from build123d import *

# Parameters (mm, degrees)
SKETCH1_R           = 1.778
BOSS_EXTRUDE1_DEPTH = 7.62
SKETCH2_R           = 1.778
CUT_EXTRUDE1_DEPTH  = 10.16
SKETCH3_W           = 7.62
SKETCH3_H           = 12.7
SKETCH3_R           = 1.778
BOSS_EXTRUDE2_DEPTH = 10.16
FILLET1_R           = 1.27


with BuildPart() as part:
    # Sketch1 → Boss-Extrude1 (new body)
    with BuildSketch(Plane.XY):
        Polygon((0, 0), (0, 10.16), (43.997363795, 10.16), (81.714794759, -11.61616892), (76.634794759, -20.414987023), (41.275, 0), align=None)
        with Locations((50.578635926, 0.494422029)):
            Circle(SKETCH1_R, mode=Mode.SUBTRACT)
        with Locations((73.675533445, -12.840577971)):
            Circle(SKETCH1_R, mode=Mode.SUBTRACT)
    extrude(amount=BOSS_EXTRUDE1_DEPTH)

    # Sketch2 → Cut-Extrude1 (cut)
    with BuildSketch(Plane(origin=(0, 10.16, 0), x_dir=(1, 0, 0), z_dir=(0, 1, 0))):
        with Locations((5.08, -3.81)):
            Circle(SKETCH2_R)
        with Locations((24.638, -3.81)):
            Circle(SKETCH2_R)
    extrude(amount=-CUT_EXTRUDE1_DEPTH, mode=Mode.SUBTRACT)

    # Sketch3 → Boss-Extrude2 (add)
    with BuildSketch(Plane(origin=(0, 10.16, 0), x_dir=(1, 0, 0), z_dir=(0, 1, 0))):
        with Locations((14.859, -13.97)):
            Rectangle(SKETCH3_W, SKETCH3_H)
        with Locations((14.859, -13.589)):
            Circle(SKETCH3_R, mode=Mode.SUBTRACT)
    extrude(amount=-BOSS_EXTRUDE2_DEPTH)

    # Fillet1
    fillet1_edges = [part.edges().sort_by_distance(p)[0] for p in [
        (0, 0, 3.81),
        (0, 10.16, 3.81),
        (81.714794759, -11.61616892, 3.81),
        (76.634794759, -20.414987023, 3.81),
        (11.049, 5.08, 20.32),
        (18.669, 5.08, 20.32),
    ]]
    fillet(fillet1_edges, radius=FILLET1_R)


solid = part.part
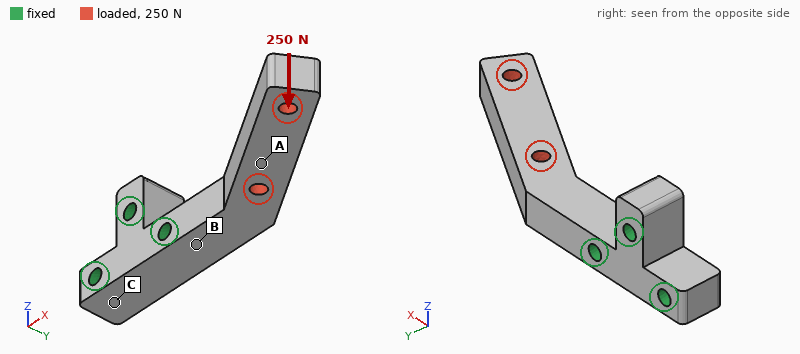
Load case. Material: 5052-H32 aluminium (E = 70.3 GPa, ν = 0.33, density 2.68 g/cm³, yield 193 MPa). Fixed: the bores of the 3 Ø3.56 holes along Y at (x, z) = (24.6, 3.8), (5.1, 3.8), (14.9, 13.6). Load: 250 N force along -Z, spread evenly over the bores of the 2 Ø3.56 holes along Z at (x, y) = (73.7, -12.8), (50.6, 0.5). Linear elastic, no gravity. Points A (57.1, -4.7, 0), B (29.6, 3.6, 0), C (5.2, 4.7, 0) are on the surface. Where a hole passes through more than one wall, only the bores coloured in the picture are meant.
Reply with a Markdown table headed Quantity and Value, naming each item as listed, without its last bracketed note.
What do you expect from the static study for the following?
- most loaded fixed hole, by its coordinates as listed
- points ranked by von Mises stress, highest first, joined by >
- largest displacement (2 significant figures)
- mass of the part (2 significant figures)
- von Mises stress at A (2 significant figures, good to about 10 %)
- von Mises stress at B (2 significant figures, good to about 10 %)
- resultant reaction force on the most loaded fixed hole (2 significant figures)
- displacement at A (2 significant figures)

| Quantity | Value |
|---|---|
| most loaded fixed hole, by its coordinates as listed | (24.6, 3.8) |
| points ranked by von Mises stress, highest first, joined by > | B > A > C |
| largest displacement | 0.40 mm |
| mass of the part | 19 g |
| von Mises stress at A | 23 MPa |
| von Mises stress at B | 88 MPa |
| resultant reaction force on the most loaded fixed hole | 450 N |
| displacement at A | 0.18 mm |
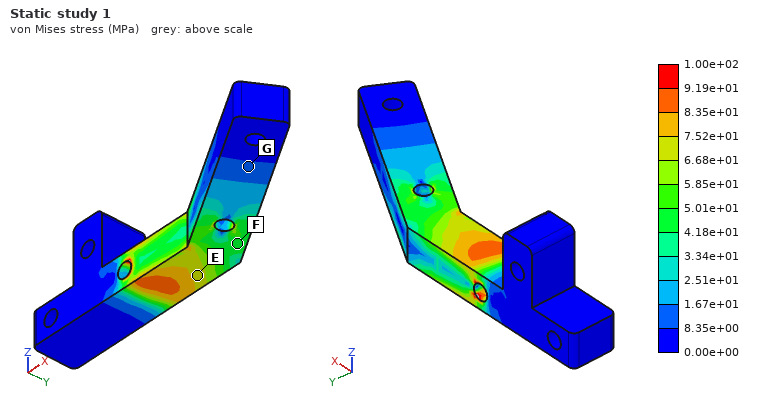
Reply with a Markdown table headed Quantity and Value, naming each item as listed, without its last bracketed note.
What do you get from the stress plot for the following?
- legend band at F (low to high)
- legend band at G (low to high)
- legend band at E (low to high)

| Quantity | Value |
|---|---|
| legend band at F | 4.18e+01 to 5.01e+01 MPa |
| legend band at G | 8.35e+00 to 1.67e+01 MPa |
| legend band at E | 6.68e+01 to 7.52e+01 MPa |
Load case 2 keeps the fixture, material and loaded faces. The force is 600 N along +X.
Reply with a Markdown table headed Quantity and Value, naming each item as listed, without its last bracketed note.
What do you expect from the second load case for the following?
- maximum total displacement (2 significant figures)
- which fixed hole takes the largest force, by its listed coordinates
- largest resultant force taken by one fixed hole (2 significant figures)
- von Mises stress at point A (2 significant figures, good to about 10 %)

| Quantity | Value |
|---|---|
| maximum total displacement | 0.19 mm |
| which fixed hole takes the largest force, by its listed coordinates | (24.6, 3.8) |
| largest resultant force taken by one fixed hole | 590 N |
| von Mises stress at point A | 9.7 MPa |
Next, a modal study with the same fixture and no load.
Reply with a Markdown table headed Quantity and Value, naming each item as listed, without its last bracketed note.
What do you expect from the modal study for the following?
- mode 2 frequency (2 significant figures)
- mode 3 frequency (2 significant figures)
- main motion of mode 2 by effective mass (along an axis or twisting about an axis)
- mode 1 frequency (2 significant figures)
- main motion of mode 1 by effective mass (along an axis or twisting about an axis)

| Quantity | Value |
|---|---|
| mode 2 frequency | 2400 Hz |
| mode 3 frequency | 9100 Hz |
| main motion of mode 2 by effective mass | along Y |
| mode 1 frequency | 1700 Hz |
| main motion of mode 1 by effective mass | along Z |
